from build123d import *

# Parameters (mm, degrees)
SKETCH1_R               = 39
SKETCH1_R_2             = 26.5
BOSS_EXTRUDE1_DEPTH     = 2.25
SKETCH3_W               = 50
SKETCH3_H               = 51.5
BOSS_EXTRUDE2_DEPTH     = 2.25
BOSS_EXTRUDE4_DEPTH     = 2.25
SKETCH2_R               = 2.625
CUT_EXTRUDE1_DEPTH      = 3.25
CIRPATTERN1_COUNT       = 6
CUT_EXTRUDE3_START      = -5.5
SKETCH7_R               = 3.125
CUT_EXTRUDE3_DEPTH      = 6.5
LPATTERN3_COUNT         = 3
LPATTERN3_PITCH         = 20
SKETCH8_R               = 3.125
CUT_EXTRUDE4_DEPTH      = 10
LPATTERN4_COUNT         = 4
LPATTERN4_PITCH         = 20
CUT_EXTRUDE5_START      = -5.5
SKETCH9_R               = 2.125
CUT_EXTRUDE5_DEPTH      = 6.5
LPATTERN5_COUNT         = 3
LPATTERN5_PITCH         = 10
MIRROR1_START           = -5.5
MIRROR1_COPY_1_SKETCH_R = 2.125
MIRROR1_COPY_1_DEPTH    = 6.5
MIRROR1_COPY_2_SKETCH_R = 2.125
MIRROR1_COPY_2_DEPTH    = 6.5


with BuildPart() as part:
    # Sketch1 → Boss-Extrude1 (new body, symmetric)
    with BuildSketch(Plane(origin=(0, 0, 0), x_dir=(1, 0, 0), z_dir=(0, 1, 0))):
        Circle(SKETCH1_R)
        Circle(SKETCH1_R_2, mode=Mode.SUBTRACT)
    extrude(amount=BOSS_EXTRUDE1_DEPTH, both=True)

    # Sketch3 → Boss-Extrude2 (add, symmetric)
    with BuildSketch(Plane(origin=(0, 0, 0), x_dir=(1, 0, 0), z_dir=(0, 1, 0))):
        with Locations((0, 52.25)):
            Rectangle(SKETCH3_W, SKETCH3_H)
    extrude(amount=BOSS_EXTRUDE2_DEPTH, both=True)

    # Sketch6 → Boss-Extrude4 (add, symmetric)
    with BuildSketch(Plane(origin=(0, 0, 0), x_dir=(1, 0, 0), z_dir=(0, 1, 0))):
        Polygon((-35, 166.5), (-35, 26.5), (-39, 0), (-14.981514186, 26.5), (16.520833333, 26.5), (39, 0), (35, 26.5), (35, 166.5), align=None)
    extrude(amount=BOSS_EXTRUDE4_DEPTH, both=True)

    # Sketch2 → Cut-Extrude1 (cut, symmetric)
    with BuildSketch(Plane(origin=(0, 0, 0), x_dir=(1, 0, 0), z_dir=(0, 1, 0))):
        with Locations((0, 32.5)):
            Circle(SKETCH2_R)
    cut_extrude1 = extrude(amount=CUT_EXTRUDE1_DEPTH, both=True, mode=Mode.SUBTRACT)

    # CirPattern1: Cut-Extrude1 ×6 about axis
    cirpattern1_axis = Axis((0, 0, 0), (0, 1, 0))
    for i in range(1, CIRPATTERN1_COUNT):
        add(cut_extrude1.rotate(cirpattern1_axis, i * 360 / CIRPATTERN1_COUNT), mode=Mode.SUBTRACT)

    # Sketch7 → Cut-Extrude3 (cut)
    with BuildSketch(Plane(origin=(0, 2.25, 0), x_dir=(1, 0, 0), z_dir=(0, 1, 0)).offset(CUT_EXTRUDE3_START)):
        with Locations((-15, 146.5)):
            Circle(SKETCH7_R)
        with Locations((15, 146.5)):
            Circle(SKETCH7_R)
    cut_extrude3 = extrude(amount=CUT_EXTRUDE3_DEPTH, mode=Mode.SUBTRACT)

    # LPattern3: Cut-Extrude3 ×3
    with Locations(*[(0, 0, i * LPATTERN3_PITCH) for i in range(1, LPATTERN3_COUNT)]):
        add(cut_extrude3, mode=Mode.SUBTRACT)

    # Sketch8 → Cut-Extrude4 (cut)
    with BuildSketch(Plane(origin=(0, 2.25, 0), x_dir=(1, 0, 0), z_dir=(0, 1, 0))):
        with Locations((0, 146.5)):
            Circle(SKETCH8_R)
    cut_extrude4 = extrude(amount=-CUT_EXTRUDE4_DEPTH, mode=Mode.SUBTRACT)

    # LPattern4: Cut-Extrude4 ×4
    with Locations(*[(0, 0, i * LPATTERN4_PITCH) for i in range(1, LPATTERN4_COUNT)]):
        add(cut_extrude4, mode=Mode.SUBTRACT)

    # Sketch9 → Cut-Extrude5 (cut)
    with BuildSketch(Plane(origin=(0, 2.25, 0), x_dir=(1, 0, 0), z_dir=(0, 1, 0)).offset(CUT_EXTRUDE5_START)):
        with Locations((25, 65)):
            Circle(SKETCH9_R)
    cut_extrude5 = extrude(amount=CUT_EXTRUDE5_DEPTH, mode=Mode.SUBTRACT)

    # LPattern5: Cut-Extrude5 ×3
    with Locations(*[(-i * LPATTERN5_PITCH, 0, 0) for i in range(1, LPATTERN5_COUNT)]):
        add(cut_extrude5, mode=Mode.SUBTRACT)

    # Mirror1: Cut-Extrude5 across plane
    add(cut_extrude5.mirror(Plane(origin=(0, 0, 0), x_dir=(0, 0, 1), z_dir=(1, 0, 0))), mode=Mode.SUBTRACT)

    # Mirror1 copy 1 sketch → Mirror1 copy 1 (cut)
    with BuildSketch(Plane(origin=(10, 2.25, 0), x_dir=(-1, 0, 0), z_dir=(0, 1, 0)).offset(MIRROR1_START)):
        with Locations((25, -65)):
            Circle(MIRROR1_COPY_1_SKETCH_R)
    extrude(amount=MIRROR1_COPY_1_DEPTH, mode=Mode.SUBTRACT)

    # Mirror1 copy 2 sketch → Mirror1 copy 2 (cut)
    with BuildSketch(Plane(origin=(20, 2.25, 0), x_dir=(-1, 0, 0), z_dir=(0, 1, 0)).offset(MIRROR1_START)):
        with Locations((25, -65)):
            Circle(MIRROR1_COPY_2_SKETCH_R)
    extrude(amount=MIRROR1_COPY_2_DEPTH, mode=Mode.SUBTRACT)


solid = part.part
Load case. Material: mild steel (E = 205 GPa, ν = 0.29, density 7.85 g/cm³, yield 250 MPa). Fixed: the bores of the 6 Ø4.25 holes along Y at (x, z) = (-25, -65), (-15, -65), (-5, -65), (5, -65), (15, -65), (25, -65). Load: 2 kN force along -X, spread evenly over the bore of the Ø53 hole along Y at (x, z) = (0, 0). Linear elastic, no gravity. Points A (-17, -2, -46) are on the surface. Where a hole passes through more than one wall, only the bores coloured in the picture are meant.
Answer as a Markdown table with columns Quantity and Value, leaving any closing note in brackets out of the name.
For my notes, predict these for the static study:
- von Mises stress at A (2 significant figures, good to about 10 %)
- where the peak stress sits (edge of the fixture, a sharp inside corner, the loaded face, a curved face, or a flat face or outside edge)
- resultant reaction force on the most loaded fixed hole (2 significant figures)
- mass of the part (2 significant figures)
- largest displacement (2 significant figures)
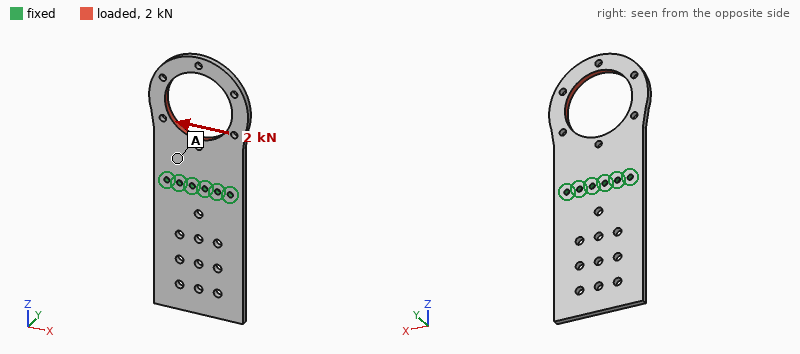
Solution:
| Quantity | Value |
|---|---|
| von Mises stress at A | 12 MPa |
| where the peak stress sits | the loaded face |
| resultant reaction force on the most loaded fixed hole | 2.1 kN |
| mass of the part | 400 g |
| largest displacement | 68 µm |
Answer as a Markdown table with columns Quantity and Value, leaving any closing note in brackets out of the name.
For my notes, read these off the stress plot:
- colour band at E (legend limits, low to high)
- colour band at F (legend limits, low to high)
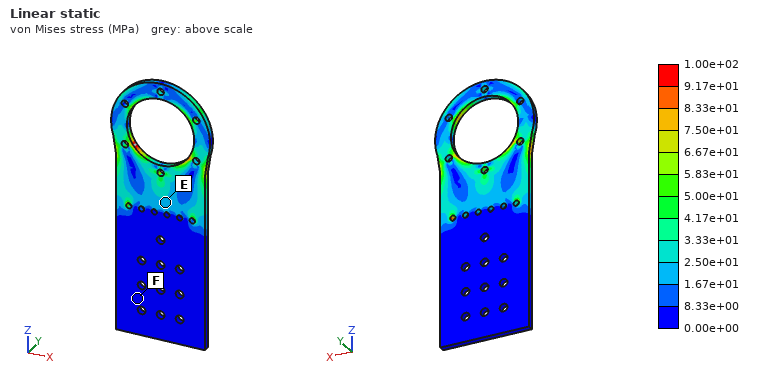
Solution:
| Quantity | Value |
|---|---|
| colour band at E | 1.67e+01 to 2.50e+01 MPa |
| colour band at F | 0.00e+00 to 8.33e+00 MPa |
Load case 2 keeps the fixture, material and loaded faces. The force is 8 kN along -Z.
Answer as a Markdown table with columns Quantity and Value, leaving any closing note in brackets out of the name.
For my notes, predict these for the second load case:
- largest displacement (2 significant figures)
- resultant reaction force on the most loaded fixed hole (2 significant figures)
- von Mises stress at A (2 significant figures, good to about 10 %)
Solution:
| Quantity | Value |
|---|---|
| largest displacement | 47 µm |
| resultant reaction force on the most loaded fixed hole | 2.2 kN |
| von Mises stress at A | 24 MPa |
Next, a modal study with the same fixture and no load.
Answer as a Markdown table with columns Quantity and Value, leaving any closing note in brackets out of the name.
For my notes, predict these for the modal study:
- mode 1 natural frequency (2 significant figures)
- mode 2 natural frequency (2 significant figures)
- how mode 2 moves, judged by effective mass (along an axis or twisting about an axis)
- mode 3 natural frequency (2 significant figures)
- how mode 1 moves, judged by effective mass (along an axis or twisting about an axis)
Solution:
| Quantity | Value |
|---|---|
| mode 1 natural frequency | 370 Hz |
| mode 2 natural frequency | 450 Hz |
| how mode 2 moves, judged by effective mass | along Y |
| mode 3 natural frequency | 1100 Hz |
| how mode 1 moves, judged by effective mass | along Y |
